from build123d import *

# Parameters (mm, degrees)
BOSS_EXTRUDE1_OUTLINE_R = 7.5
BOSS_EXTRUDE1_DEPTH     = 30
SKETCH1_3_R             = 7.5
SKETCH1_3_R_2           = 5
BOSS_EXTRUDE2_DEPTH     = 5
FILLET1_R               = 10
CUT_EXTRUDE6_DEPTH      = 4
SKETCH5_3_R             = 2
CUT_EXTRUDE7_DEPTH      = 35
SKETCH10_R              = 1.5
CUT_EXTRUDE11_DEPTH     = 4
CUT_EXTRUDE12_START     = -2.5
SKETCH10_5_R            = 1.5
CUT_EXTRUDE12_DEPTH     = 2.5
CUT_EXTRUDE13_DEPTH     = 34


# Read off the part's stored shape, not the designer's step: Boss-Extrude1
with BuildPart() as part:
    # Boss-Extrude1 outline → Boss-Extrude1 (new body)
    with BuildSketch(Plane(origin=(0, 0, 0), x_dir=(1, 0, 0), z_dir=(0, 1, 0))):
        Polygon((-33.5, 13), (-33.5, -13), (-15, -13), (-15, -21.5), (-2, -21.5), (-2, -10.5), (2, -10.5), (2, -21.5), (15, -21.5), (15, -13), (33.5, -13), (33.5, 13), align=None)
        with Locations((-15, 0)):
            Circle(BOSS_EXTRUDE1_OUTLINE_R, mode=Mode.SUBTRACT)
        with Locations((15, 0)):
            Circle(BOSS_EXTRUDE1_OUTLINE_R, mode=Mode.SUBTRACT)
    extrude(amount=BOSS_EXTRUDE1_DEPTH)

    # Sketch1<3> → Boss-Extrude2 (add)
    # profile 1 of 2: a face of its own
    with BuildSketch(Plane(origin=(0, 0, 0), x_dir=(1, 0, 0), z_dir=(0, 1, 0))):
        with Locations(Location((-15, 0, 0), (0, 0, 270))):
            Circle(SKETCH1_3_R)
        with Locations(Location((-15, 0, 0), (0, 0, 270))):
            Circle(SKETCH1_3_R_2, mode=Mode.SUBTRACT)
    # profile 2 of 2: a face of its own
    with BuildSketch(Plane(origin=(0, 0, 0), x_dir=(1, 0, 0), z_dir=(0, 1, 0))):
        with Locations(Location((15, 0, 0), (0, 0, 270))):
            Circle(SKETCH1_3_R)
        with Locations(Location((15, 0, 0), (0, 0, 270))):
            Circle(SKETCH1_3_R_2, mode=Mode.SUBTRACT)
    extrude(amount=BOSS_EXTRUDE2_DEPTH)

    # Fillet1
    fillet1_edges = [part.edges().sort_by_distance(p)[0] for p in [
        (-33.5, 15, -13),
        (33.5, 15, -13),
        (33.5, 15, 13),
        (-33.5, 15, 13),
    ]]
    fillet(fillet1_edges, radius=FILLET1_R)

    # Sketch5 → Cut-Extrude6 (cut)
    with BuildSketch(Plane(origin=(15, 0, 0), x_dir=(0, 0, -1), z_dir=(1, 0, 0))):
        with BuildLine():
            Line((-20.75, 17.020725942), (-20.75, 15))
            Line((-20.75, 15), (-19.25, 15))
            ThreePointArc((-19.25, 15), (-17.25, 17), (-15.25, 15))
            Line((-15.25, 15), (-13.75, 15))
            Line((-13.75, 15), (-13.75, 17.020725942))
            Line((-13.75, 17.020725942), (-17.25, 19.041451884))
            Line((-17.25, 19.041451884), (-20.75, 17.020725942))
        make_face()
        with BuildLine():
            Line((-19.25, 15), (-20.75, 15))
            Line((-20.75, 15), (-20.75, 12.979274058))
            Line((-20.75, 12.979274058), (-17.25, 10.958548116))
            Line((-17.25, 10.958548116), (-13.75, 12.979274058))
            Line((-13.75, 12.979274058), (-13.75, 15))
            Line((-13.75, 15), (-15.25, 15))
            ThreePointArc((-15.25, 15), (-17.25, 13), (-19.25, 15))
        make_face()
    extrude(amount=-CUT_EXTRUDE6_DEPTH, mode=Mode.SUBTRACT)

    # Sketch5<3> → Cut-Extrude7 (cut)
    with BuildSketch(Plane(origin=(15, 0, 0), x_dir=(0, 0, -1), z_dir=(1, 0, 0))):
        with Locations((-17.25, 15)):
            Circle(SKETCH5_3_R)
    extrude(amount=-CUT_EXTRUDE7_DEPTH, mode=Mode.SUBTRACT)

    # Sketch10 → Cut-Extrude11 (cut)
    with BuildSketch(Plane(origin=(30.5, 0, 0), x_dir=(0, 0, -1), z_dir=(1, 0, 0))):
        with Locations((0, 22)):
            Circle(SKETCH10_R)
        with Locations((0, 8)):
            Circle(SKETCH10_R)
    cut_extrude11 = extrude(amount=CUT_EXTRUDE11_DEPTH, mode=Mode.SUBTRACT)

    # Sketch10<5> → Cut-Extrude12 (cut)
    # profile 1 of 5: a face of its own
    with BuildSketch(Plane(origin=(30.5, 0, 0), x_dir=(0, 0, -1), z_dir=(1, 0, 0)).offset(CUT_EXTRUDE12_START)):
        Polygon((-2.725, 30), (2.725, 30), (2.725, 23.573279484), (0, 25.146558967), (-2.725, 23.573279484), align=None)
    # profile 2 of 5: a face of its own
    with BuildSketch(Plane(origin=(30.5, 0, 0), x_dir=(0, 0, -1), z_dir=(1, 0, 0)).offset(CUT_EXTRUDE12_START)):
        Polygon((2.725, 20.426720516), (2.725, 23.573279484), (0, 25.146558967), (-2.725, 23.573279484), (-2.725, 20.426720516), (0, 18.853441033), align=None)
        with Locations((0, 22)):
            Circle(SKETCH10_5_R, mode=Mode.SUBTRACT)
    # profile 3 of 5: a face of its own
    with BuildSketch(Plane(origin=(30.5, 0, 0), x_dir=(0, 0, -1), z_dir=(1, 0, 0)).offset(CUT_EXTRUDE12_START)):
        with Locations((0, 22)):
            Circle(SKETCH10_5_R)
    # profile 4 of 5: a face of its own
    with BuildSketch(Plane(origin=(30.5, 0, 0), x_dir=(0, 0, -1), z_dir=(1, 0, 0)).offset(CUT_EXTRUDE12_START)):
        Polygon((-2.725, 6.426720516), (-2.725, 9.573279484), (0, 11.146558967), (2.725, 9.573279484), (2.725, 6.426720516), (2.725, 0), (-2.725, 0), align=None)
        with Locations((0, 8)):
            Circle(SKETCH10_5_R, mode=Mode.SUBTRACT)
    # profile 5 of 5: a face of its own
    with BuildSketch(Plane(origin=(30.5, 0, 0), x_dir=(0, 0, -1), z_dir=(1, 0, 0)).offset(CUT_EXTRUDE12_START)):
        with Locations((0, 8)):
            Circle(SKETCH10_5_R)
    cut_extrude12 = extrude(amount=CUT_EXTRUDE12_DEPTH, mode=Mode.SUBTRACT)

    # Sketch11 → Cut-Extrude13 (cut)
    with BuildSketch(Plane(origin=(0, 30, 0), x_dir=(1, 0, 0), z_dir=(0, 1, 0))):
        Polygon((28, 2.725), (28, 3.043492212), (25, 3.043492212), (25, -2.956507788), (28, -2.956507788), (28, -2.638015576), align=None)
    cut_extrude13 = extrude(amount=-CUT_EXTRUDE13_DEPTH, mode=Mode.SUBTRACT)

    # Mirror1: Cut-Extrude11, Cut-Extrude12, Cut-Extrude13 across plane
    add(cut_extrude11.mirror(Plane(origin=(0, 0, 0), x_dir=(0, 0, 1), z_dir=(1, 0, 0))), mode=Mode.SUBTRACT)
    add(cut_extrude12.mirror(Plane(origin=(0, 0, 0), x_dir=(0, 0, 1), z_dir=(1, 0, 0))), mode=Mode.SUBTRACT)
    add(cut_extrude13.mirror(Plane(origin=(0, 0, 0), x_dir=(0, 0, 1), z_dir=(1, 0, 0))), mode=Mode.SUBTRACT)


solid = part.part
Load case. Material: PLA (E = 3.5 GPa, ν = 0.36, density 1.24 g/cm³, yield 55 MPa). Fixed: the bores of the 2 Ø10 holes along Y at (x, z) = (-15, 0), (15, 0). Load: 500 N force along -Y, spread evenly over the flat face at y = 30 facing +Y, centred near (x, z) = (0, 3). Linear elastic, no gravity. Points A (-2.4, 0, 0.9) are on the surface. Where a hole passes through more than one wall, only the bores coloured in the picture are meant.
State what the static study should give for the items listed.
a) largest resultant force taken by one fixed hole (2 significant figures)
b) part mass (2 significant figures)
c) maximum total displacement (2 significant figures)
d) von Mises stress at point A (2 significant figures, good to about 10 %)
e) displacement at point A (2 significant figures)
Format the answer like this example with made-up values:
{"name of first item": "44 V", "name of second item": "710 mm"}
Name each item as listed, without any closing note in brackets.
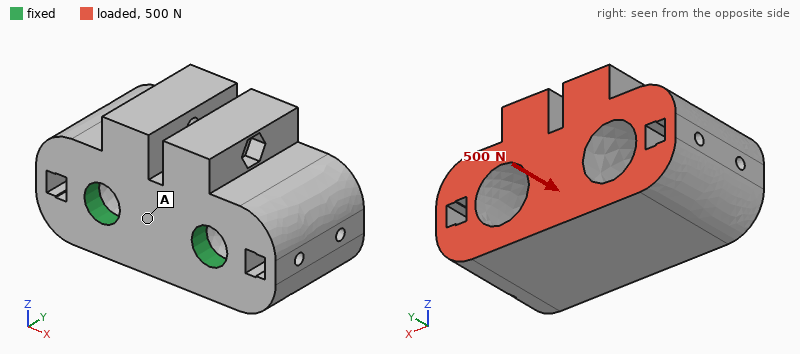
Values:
{"largest resultant force taken by one fixed hole": "250 N", "part mass": "55 g", "maximum total displacement": "27 µm", "von Mises stress at point A": "0.69 MPa", "displacement at point A": "6.4 µm"}
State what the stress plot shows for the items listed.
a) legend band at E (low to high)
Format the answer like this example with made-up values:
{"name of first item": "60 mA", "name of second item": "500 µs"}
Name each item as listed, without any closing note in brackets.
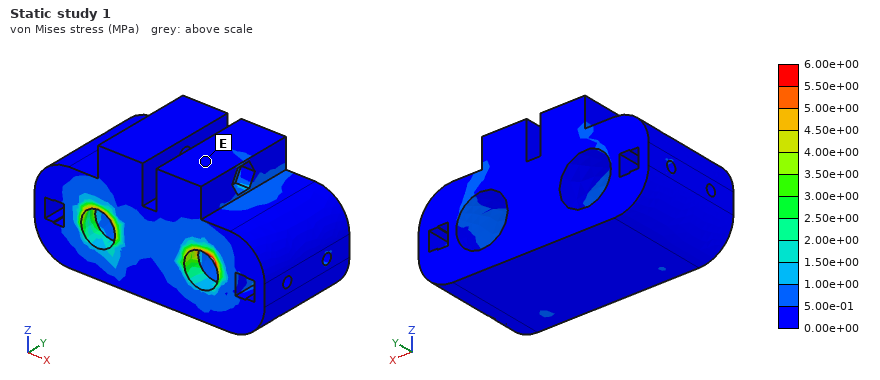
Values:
{"legend band at E": "0.00e+00 to 5.00e-01 MPa"}
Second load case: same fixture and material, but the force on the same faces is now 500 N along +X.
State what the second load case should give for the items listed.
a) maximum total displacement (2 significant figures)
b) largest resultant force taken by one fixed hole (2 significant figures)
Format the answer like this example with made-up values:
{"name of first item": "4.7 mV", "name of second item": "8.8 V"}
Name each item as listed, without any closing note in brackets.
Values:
{"maximum total displacement": "56 µm", "largest resultant force taken by one fixed hole": "480 N"}
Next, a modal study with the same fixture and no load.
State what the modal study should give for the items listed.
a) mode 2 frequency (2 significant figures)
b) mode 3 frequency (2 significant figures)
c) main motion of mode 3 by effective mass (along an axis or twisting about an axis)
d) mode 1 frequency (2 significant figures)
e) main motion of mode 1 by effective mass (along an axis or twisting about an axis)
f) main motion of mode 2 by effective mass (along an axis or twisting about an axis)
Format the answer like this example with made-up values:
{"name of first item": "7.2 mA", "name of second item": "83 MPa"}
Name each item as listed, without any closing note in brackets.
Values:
{"mode 2 frequency": "3400 Hz", "mode 3 frequency": "3900 Hz", "main motion of mode 3 by effective mass": "twisting about Y", "mode 1 frequency": "1800 Hz", "main motion of mode 1 by effective mass": "along Z", "main motion of mode 2 by effective mass": "along X"}
